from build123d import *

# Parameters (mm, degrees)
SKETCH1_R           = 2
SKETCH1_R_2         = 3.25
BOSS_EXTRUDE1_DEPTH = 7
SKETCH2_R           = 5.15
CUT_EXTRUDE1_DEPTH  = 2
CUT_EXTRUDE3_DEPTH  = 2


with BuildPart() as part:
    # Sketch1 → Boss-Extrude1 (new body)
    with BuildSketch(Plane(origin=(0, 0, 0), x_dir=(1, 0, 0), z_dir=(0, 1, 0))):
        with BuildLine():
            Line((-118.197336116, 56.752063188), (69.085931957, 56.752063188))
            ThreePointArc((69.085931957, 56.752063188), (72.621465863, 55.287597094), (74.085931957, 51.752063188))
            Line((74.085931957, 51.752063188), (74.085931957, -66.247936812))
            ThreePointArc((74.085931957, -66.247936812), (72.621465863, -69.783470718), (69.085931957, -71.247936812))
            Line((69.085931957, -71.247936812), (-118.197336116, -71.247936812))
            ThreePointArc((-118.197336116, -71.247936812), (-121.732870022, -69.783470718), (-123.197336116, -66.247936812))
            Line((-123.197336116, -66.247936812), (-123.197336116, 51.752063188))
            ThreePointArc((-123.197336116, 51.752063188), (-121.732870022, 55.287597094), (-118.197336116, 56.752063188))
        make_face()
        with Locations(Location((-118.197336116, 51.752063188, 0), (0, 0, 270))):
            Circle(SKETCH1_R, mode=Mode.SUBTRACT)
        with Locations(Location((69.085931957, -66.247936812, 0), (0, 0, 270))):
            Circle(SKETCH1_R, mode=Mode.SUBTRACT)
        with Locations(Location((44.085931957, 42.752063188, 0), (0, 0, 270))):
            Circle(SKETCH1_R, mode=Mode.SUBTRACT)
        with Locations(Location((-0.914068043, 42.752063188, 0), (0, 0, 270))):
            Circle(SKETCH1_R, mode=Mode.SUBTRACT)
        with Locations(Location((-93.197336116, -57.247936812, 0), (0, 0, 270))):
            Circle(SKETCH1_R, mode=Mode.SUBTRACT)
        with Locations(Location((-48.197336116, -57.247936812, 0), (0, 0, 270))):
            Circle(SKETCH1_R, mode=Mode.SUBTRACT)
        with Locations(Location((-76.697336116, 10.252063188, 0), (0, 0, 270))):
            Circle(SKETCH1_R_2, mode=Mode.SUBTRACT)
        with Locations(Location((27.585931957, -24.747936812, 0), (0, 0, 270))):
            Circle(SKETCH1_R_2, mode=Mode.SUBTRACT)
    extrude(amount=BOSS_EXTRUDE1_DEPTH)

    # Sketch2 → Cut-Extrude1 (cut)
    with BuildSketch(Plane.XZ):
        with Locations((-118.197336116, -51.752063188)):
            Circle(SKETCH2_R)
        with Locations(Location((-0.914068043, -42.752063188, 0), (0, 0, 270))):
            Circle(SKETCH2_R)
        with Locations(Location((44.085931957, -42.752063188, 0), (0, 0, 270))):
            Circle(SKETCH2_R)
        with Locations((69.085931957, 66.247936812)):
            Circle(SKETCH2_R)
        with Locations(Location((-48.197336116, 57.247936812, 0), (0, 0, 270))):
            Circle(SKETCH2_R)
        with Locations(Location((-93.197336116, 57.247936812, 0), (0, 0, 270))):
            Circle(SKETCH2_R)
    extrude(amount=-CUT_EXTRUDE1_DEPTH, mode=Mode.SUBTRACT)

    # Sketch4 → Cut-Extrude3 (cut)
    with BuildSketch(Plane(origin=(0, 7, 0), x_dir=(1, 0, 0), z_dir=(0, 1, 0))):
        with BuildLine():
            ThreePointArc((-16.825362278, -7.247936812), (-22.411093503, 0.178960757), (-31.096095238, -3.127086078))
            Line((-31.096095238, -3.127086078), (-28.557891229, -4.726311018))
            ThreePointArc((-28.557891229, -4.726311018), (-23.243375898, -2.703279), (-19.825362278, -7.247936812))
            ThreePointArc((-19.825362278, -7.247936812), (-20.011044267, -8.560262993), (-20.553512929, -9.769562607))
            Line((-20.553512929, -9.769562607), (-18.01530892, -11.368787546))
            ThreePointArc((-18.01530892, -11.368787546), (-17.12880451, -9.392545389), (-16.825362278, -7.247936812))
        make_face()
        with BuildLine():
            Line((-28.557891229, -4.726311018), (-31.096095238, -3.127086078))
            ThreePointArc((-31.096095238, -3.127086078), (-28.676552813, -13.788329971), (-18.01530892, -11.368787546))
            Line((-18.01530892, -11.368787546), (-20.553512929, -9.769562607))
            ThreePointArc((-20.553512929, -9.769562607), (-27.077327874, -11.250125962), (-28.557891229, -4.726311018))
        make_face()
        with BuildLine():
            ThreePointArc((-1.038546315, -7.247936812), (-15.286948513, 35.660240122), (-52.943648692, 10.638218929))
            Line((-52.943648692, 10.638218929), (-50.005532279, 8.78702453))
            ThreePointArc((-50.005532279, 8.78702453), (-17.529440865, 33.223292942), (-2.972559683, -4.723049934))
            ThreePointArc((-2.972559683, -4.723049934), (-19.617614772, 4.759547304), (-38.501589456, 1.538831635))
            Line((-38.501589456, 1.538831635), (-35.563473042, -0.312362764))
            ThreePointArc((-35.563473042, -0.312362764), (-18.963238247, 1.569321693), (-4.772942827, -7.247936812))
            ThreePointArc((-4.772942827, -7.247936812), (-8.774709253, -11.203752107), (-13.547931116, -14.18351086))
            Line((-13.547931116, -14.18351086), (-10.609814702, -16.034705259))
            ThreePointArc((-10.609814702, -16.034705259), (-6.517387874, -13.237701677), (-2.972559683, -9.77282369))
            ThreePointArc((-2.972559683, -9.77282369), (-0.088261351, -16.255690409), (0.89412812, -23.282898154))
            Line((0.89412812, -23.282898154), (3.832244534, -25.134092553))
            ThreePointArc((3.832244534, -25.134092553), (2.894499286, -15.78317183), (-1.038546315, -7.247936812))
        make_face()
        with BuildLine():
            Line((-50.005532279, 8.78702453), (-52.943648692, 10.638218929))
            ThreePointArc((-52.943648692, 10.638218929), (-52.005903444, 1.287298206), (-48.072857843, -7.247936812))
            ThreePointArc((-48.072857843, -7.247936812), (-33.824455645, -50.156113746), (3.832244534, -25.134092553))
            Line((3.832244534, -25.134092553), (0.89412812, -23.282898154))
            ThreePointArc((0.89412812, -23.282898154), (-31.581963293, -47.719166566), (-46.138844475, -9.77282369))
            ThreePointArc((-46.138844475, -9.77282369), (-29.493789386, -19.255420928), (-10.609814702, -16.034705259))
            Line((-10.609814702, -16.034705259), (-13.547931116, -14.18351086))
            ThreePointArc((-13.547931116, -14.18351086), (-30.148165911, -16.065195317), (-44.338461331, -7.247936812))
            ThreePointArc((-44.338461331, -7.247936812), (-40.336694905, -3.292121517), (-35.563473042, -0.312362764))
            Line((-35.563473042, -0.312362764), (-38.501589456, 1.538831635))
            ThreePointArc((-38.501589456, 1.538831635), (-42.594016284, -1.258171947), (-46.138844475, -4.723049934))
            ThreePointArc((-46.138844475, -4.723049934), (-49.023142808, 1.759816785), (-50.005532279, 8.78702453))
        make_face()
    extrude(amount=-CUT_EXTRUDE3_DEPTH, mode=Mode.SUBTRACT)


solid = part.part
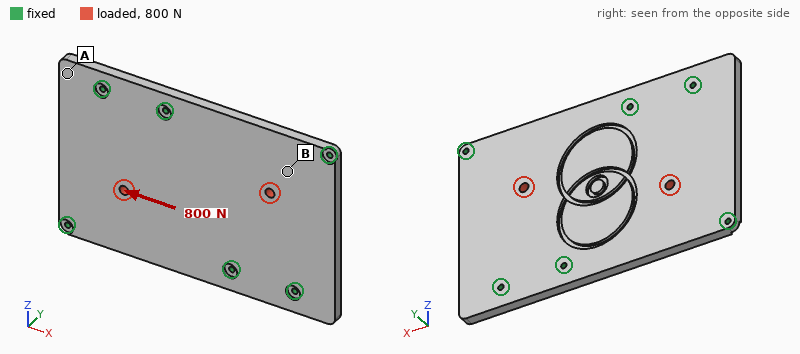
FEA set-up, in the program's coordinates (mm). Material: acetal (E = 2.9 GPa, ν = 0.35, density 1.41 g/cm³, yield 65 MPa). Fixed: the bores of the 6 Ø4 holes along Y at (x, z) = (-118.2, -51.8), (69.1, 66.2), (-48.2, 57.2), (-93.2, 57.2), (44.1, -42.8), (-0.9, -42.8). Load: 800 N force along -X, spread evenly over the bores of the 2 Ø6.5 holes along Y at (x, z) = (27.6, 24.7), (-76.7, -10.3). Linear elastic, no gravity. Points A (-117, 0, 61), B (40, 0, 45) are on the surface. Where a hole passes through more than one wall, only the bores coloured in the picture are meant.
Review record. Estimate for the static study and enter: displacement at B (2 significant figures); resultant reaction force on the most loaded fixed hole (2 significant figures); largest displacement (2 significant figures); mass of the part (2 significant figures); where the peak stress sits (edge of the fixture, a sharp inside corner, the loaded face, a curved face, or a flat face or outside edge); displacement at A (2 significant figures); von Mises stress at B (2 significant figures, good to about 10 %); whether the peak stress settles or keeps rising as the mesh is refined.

18 µm
180 N
32 µm
240 g
edge of the fixture
9.9 µm
0.78 MPa
keeps rising
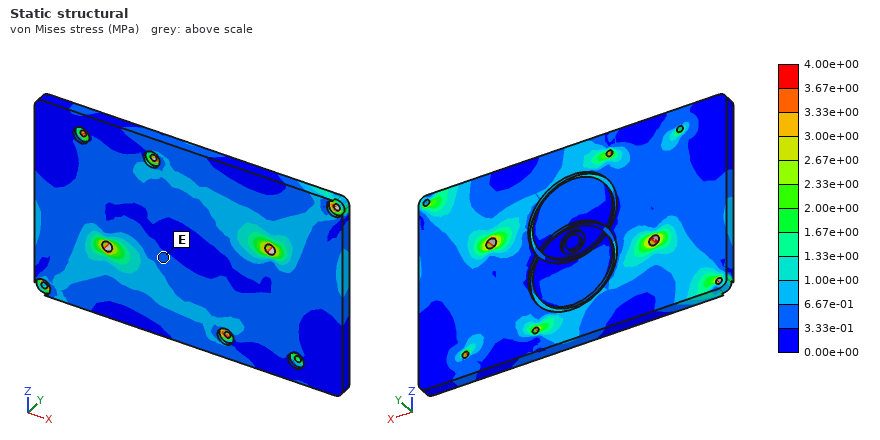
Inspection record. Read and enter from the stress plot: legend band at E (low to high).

3.33e-01 to 6.67e-01 MPa
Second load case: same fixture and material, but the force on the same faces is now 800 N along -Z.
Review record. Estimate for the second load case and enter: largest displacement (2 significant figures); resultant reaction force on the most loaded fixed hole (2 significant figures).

29 µm
150 N
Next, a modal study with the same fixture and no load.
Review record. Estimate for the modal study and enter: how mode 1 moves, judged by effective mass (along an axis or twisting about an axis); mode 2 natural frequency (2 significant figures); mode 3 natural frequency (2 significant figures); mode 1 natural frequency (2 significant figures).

along Y
550 Hz
740 Hz
510 Hz
